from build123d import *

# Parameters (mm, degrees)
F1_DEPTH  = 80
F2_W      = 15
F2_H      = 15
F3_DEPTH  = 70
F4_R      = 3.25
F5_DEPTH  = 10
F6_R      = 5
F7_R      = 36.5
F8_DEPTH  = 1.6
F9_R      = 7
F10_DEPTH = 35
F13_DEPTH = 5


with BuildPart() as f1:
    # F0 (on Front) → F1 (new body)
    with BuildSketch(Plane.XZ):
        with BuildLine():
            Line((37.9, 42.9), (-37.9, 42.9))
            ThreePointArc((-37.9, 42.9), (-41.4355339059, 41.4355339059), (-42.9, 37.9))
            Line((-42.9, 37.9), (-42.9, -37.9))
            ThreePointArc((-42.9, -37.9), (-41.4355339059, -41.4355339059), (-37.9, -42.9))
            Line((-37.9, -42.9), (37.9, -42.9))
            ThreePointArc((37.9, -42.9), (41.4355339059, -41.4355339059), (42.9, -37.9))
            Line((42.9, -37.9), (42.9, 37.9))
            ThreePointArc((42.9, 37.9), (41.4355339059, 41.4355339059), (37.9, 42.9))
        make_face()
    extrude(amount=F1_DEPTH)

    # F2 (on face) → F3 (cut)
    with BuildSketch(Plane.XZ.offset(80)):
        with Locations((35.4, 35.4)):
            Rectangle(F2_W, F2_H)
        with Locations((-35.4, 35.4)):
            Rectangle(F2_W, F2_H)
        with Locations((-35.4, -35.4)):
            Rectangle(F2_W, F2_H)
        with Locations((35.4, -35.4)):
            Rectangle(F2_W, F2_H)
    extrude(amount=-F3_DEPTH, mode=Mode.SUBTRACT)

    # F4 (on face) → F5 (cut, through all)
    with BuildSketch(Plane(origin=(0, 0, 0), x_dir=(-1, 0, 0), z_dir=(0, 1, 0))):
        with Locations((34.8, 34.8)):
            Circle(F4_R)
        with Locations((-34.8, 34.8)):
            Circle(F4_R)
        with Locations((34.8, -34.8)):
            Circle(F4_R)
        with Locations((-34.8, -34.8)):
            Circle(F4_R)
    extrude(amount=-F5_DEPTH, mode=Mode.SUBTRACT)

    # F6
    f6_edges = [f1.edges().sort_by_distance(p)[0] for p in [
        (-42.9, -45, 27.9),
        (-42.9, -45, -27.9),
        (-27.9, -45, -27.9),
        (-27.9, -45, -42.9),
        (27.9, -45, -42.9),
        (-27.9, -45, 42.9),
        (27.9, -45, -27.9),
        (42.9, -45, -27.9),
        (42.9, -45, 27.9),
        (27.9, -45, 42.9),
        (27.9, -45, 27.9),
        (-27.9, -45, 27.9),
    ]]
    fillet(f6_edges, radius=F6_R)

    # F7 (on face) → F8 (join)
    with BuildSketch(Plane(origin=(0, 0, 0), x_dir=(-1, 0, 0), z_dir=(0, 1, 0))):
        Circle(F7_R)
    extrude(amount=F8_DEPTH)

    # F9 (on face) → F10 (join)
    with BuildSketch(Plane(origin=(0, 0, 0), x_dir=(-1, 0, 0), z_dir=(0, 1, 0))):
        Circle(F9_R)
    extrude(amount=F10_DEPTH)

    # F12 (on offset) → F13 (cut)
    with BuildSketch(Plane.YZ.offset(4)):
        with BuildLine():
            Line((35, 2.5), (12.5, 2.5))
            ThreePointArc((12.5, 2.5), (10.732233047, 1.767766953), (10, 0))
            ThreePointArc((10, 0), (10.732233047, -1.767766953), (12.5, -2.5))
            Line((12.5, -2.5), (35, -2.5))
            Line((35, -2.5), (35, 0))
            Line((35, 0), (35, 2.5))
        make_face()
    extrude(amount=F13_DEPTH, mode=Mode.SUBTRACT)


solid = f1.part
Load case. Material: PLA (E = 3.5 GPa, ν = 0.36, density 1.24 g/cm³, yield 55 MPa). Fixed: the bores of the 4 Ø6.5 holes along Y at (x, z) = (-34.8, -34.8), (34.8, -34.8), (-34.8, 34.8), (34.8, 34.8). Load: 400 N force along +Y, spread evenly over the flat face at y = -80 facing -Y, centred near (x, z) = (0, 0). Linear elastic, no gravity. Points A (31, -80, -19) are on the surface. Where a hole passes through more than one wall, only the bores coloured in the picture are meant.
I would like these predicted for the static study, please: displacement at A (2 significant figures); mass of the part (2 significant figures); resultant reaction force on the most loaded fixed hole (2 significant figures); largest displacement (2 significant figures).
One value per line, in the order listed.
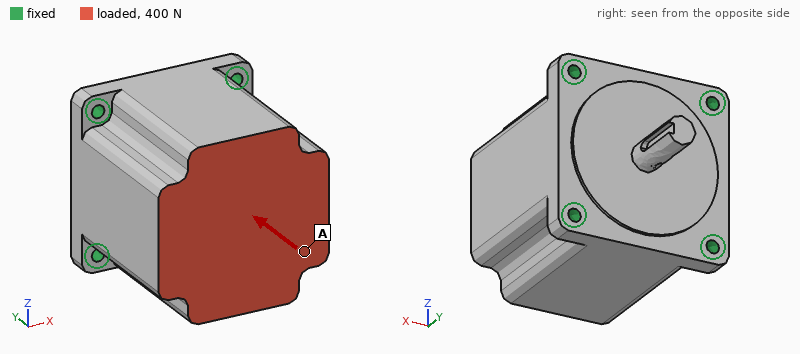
5.6 µm
660 g
110 N
5.6 µm
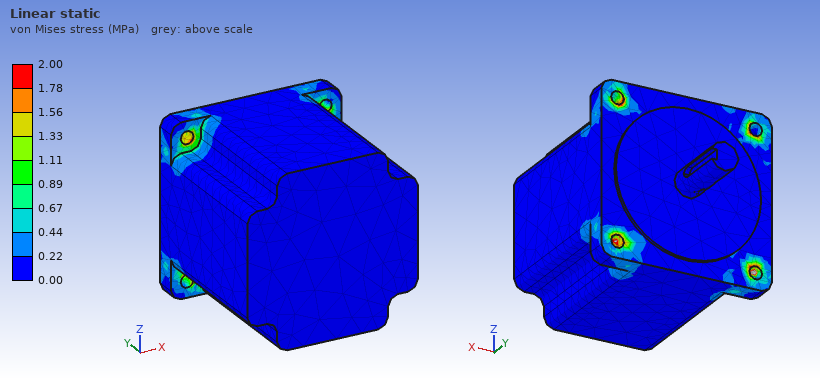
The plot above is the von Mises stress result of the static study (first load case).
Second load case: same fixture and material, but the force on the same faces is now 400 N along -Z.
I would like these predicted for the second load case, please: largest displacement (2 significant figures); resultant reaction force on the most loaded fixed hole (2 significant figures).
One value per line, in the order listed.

34 µm
260 N
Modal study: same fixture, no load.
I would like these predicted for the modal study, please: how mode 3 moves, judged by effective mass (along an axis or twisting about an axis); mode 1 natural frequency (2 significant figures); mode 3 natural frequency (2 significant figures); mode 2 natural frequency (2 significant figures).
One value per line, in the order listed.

along Y
1200 Hz
1800 Hz
1200 Hz
